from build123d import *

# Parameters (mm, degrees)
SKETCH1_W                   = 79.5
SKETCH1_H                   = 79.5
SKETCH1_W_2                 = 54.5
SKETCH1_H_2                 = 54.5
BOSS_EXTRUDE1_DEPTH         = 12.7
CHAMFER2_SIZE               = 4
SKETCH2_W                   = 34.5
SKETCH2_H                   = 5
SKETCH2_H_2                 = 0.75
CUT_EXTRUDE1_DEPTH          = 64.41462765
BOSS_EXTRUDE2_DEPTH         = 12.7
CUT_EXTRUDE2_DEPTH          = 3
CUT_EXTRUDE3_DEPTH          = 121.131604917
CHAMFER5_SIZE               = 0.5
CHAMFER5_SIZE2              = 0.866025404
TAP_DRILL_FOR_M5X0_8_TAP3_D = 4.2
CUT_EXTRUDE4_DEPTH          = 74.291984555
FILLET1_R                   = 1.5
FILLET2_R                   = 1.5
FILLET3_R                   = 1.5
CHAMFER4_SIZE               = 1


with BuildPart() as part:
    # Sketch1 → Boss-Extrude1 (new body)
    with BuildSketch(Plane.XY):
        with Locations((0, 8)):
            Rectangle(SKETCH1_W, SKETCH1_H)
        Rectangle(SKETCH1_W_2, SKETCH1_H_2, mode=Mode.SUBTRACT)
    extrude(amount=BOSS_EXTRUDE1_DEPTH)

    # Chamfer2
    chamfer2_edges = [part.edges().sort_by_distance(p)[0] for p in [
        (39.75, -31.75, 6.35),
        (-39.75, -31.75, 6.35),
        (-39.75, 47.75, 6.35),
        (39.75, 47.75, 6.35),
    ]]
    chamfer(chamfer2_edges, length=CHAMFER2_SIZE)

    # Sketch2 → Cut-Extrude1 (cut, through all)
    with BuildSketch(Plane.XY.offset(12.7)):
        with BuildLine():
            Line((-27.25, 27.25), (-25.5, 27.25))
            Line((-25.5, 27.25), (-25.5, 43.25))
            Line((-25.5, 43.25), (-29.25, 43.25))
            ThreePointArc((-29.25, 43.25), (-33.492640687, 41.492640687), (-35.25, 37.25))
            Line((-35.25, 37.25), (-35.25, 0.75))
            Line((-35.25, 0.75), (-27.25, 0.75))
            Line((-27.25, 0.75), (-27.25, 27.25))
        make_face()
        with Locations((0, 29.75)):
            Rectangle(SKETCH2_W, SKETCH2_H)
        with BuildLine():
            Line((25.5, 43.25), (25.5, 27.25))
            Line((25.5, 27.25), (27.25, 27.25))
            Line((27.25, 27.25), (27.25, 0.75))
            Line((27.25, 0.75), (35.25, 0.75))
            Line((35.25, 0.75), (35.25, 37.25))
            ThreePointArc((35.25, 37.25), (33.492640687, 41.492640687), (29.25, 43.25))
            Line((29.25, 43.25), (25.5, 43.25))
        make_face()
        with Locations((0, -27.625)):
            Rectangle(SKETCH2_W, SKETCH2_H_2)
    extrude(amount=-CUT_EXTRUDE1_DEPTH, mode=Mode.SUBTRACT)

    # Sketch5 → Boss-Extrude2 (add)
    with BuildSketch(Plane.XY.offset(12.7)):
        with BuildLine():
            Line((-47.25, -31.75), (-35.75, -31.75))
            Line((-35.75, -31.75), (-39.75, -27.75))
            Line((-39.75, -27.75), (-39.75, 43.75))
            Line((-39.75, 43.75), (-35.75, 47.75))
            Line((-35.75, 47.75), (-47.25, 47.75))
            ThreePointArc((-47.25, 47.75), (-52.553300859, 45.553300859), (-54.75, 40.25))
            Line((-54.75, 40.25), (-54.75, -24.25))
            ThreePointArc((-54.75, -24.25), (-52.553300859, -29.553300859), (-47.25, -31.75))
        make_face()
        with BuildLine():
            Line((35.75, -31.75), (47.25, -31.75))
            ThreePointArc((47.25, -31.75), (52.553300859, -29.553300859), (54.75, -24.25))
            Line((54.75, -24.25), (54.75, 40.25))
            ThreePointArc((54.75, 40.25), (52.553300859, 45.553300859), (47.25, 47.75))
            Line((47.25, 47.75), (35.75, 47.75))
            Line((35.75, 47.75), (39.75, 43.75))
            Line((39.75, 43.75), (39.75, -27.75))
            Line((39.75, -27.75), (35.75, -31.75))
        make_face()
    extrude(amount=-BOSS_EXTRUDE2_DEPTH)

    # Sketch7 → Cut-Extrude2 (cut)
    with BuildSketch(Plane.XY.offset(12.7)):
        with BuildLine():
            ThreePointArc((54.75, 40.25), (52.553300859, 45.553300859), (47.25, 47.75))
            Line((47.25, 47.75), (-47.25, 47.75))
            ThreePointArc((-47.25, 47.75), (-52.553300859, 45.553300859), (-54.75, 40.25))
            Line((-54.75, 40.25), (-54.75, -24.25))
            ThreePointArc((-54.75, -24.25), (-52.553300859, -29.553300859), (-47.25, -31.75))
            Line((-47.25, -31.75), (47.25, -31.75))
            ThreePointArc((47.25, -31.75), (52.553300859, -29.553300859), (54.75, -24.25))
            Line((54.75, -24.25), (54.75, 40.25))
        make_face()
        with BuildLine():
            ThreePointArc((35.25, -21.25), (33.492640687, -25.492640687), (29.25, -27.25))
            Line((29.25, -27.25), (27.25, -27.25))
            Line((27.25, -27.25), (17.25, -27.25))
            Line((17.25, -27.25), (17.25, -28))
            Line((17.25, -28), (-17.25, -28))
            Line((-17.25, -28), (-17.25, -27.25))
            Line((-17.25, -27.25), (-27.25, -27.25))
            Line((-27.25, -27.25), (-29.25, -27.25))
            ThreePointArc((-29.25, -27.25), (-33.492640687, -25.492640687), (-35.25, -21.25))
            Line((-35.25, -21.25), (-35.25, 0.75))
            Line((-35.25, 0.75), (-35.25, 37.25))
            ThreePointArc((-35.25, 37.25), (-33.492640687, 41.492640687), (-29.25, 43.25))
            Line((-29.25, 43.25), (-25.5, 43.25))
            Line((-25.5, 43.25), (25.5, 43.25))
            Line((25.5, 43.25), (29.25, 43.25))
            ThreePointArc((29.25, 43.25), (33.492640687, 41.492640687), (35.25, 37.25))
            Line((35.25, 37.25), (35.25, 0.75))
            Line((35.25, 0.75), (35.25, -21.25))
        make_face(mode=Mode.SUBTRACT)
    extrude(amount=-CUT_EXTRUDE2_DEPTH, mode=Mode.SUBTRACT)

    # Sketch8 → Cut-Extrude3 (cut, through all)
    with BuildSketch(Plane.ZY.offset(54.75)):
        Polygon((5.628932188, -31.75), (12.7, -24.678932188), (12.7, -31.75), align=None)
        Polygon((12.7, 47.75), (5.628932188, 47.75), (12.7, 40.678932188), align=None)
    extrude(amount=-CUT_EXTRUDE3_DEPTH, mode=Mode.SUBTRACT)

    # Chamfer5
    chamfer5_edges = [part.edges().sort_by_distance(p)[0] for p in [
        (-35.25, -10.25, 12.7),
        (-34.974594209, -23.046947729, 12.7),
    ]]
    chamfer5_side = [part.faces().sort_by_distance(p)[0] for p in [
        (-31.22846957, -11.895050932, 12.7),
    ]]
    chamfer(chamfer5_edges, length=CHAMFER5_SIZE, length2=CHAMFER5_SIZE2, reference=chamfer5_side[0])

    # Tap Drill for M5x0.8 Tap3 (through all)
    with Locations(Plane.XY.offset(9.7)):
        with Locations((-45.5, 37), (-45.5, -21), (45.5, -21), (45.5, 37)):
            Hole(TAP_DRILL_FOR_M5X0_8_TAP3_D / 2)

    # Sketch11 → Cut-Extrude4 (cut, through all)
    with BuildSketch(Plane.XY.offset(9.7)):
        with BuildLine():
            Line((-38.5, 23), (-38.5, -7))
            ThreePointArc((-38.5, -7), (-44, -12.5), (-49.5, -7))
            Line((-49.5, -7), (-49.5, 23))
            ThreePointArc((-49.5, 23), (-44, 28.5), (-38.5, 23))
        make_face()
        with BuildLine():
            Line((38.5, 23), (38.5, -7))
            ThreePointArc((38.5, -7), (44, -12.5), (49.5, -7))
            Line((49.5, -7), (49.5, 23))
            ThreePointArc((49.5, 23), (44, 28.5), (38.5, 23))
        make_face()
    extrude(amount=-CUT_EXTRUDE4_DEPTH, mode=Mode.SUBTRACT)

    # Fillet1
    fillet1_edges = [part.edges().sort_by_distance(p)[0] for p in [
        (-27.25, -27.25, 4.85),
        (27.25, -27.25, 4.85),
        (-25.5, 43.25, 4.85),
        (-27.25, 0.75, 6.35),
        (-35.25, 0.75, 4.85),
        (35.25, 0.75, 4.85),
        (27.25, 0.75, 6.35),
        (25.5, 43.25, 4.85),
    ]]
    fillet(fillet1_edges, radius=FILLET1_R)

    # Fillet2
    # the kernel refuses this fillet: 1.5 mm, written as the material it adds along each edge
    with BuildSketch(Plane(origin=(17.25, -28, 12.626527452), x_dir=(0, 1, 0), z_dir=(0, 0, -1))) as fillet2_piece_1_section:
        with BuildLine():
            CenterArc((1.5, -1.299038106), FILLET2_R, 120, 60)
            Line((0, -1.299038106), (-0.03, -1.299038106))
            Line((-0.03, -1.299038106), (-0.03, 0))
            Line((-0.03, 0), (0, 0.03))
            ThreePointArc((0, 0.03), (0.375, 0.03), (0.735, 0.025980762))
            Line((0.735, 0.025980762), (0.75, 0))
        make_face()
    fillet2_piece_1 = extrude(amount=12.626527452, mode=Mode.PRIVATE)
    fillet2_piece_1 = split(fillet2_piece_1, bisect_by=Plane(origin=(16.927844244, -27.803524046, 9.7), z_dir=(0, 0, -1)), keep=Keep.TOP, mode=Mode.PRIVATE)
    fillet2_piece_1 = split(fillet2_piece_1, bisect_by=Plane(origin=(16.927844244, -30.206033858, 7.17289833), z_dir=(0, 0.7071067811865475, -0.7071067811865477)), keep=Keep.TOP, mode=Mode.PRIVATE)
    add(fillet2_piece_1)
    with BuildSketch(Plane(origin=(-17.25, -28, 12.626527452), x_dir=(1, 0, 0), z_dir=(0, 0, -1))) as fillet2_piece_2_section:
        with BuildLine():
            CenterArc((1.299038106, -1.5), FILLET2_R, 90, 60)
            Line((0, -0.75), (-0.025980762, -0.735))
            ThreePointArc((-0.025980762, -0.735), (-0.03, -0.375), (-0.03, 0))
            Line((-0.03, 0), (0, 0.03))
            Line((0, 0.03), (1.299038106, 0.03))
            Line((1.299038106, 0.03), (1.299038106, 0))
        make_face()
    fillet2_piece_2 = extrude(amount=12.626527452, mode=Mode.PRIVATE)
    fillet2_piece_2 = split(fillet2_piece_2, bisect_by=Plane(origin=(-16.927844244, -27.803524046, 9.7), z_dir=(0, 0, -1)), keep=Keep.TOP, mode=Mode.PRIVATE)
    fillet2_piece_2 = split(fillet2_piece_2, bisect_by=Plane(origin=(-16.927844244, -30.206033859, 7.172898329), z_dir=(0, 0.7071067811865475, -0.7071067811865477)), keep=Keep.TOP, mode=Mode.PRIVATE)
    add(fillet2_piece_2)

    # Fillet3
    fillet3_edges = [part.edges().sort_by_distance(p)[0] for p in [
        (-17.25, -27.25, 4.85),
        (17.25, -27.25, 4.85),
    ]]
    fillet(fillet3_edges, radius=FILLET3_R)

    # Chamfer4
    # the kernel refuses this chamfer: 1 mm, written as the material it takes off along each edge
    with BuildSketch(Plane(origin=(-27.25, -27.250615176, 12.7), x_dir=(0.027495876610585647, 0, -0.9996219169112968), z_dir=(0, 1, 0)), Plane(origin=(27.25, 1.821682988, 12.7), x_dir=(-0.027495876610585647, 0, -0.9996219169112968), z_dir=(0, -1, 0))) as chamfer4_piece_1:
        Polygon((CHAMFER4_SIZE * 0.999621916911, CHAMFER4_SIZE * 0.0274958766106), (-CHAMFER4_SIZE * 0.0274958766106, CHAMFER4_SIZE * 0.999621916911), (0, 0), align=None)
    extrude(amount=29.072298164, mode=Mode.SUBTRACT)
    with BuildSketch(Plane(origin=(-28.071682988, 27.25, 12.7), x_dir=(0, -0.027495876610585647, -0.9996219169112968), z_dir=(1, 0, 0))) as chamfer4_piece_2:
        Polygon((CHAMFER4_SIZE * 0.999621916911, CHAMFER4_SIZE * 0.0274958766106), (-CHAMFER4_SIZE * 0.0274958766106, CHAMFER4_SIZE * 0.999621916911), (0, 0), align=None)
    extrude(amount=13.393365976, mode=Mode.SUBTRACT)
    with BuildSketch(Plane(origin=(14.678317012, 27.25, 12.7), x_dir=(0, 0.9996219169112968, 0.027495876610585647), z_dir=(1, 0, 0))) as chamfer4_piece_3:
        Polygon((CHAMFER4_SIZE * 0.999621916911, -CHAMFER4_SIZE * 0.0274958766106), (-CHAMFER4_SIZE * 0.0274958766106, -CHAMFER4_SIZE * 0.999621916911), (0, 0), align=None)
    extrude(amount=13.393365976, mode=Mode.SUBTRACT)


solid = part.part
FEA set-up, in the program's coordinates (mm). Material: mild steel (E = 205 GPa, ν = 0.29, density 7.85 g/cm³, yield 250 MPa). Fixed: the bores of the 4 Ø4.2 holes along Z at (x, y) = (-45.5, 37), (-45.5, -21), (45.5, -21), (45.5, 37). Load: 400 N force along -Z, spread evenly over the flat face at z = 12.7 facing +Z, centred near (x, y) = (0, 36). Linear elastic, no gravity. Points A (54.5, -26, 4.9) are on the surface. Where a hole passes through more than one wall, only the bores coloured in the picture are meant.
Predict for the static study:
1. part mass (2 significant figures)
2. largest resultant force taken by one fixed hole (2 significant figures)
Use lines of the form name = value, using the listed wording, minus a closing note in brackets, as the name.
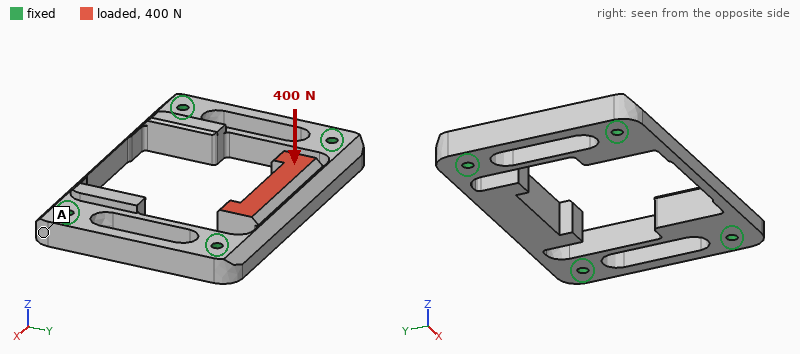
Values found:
part mass = 300 g
largest resultant force taken by one fixed hole = 200 N
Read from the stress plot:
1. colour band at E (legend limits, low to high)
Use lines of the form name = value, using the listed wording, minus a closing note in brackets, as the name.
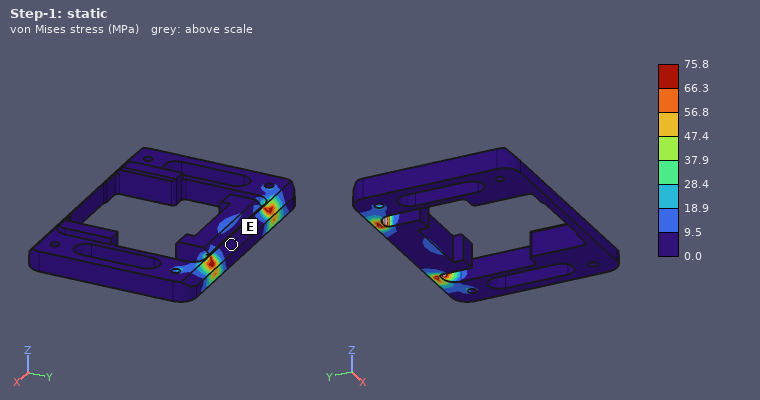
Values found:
colour band at E = 0.0 to 9.5 MPa
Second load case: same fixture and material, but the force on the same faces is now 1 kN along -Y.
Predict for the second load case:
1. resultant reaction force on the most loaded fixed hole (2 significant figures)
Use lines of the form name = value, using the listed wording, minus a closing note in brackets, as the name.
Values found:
resultant reaction force on the most loaded fixed hole = 460 N
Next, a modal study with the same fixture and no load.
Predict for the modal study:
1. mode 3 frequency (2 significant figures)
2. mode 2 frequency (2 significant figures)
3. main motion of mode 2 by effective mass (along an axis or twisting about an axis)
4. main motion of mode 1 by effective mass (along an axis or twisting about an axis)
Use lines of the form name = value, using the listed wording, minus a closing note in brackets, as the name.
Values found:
mode 3 frequency = 6200 Hz
mode 2 frequency = 5000 Hz
main motion of mode 2 by effective mass = along Y
main motion of mode 1 by effective mass = along Z
